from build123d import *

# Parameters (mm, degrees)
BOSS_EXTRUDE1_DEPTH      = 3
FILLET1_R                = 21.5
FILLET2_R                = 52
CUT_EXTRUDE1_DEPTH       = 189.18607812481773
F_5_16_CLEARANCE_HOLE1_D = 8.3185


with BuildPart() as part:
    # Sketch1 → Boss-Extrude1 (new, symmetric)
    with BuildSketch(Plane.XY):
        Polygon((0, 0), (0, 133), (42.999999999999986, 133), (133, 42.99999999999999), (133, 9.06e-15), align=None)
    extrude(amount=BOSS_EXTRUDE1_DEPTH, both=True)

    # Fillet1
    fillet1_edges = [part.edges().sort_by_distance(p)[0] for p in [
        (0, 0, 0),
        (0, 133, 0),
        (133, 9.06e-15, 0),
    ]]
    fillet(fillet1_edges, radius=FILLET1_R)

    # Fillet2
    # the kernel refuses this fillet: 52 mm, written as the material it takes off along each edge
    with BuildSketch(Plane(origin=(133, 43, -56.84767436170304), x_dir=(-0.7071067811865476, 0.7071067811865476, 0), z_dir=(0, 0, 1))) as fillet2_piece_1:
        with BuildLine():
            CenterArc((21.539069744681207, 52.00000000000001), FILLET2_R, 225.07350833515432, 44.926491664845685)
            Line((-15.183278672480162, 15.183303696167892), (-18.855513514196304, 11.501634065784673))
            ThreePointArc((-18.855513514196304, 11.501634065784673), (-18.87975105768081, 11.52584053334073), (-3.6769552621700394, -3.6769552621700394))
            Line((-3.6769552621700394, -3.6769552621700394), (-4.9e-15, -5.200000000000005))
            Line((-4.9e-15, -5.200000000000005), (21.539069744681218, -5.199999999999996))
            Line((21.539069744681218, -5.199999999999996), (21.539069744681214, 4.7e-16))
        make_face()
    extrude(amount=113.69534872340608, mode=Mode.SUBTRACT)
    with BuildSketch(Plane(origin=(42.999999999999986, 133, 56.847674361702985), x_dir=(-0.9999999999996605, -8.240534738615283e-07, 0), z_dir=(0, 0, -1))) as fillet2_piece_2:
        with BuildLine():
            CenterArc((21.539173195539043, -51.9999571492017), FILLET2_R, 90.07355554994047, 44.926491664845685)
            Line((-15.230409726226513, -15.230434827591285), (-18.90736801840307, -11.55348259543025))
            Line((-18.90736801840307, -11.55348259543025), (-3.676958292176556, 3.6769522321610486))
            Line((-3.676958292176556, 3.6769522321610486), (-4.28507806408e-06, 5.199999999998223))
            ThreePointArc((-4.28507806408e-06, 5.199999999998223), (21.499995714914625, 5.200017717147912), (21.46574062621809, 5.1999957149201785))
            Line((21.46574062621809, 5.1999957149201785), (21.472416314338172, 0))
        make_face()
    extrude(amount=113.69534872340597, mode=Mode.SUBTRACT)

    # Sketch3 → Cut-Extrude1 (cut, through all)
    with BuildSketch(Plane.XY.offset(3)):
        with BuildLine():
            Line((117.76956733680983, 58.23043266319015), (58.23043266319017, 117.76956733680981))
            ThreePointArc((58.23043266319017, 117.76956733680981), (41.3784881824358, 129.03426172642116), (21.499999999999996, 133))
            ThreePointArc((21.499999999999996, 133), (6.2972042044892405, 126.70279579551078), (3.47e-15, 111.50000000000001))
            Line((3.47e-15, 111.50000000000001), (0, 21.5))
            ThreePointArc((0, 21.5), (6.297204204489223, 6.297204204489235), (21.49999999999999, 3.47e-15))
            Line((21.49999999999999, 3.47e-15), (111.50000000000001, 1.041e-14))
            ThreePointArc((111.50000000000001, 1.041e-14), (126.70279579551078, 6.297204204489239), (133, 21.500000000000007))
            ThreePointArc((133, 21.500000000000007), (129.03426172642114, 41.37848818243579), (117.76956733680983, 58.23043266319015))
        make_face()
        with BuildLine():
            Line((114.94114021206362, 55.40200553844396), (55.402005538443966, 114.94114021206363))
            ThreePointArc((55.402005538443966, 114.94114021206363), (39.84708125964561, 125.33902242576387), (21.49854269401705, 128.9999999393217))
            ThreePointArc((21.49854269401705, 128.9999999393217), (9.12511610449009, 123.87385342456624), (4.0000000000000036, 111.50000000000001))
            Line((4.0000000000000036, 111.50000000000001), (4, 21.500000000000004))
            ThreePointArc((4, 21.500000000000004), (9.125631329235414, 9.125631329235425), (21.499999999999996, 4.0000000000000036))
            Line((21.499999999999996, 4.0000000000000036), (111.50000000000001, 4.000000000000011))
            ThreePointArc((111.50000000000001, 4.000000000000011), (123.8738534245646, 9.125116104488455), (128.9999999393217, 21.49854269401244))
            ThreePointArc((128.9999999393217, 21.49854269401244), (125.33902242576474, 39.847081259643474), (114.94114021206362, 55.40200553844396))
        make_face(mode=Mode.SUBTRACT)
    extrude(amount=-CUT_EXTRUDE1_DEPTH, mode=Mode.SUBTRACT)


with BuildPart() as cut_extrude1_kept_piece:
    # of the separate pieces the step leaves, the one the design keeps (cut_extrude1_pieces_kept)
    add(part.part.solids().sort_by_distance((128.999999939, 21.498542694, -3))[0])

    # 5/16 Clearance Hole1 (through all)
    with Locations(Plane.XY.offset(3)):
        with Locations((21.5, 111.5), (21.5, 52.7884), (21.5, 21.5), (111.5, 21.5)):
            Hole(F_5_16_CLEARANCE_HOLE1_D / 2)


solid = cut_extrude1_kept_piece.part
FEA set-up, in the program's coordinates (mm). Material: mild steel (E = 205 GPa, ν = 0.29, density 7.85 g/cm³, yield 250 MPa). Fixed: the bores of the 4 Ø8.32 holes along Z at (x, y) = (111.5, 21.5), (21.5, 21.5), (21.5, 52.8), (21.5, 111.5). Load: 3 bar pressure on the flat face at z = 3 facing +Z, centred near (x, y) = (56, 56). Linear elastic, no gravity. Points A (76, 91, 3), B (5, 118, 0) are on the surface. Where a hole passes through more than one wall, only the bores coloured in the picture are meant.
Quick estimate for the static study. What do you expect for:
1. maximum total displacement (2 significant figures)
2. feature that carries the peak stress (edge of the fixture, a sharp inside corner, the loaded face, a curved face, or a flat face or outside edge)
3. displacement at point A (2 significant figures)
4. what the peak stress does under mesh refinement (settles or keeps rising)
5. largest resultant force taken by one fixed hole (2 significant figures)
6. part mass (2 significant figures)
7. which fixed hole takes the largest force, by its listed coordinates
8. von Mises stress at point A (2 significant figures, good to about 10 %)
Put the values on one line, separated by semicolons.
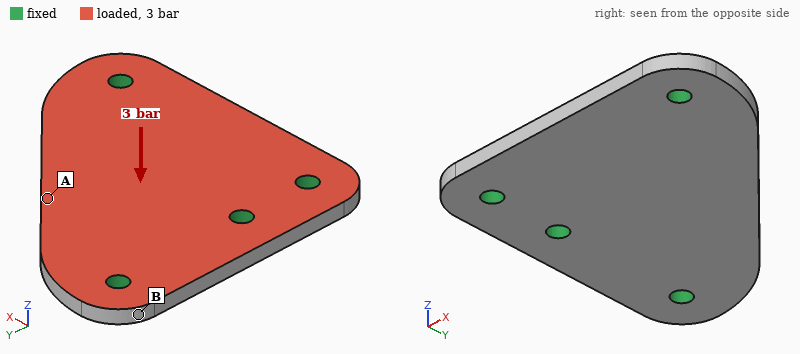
58 µm; edge of the fixture; 53 µm; keeps rising; 1.1 kN; 530 g; (111.5, 21.5); 22 MPa
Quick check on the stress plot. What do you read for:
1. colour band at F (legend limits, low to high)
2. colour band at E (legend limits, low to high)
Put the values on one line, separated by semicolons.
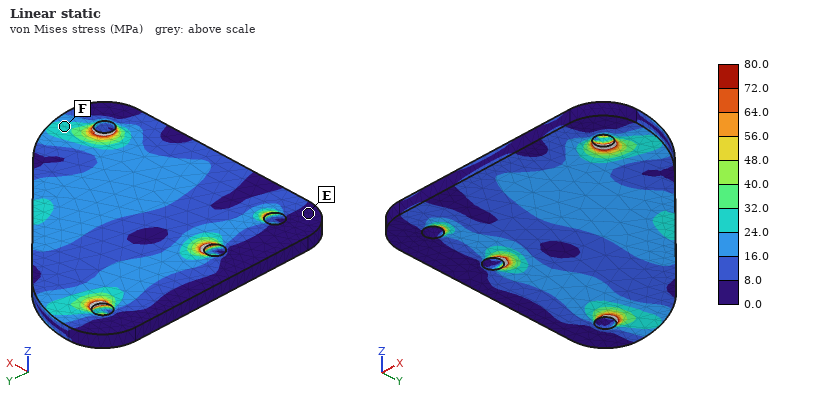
24.0 to 32.0 MPa; 0.0 to 8.0 MPa
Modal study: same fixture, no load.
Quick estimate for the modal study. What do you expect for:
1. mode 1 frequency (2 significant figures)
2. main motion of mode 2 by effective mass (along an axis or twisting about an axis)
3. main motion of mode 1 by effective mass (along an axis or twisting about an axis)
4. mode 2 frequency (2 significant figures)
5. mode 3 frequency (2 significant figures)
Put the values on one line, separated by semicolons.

2200 Hz; along Z; along Z; 4200 Hz; 5200 Hz
